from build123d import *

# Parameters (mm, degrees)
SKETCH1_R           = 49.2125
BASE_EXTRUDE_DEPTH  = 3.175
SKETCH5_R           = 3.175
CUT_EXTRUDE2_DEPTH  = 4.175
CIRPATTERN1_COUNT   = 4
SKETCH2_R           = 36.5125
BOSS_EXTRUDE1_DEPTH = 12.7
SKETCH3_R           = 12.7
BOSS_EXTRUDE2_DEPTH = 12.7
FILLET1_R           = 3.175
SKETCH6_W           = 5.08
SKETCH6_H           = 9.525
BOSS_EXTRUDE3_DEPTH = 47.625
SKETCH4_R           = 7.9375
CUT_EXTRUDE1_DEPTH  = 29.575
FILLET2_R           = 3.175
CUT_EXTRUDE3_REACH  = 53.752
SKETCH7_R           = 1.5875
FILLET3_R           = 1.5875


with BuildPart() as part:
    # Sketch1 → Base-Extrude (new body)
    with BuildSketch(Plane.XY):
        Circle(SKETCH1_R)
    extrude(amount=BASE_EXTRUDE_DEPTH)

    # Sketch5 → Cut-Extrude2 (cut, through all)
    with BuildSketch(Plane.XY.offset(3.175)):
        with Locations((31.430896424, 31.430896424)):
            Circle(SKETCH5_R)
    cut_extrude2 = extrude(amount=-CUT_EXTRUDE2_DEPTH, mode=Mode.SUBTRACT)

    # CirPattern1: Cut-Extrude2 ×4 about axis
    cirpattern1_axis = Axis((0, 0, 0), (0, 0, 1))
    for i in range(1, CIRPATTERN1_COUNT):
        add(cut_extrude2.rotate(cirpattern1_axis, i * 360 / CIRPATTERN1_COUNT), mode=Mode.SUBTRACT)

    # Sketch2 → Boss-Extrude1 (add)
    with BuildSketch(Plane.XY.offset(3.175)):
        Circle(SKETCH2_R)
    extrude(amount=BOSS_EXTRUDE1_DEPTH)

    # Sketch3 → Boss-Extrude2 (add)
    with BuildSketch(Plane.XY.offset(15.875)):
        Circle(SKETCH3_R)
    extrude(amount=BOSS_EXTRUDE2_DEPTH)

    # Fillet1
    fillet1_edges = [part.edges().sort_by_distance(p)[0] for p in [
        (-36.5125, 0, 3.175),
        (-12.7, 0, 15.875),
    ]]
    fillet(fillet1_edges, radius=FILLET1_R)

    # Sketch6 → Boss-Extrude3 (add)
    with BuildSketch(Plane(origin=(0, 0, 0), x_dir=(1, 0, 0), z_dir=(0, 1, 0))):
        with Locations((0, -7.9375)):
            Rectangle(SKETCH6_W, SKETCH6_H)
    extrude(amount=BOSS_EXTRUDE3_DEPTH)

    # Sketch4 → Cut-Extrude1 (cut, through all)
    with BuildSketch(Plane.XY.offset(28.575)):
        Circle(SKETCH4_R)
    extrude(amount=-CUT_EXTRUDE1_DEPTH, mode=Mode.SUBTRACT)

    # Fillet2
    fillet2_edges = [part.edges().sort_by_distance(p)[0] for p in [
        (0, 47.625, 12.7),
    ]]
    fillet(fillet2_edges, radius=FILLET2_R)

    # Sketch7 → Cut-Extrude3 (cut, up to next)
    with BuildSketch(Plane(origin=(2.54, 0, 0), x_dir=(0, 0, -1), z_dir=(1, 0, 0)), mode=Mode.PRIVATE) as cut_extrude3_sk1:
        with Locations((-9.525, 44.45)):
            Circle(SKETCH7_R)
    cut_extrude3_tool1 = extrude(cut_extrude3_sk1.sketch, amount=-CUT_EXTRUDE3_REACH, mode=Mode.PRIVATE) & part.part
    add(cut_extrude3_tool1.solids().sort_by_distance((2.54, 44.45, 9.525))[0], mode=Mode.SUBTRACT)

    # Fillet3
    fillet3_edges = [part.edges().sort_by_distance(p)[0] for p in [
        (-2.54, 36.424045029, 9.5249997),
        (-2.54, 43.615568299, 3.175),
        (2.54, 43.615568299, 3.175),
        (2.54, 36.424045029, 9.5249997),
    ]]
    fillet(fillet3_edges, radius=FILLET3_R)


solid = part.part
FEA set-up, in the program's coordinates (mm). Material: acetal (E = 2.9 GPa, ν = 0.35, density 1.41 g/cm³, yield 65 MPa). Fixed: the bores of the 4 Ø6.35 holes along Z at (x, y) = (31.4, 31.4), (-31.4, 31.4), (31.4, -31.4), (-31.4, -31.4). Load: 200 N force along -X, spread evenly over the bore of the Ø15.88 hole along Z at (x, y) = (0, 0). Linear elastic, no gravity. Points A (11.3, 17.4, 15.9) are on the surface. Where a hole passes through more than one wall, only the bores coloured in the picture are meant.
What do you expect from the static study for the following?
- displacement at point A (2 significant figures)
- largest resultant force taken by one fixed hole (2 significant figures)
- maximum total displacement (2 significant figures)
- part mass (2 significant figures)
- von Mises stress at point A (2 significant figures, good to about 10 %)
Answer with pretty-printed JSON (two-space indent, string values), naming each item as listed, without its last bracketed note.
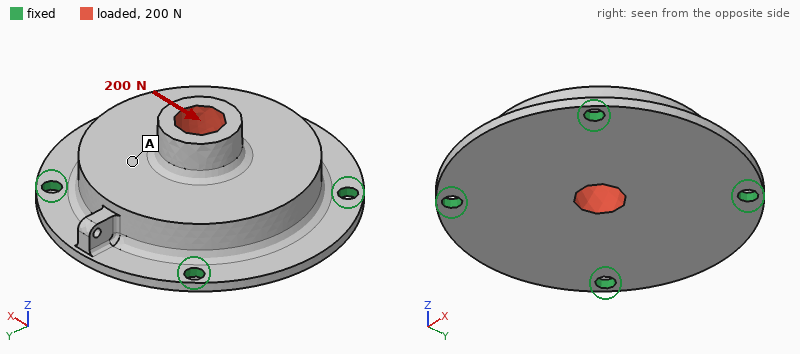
{
  "displacement at point A": "7.6 µm",
  "largest resultant force taken by one fixed hole": "58 N",
  "maximum total displacement": "17 µm",
  "part mass": "110 g",
  "von Mises stress at point A": "0.24 MPa"
}
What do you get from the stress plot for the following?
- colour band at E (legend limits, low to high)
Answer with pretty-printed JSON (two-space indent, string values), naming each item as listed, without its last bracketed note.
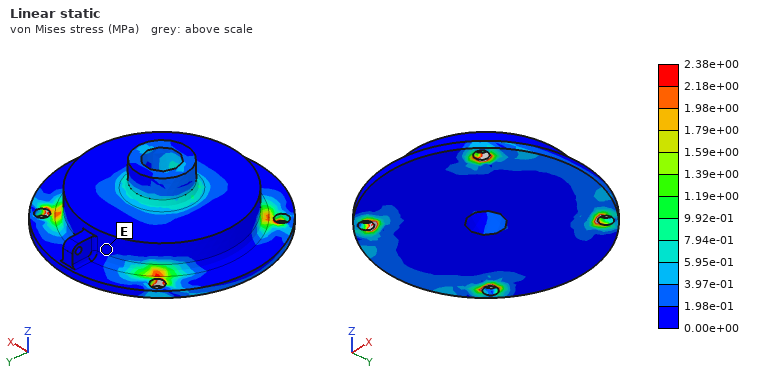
{
  "colour band at E": "0.00e+00 to 1.98e-01 MPa"
}
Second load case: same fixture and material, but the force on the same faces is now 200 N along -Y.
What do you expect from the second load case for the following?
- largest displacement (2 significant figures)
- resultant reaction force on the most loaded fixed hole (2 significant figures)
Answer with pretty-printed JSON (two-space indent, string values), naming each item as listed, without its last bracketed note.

{
  "largest displacement": "17 µm",
  "resultant reaction force on the most loaded fixed hole": "58 N"
}
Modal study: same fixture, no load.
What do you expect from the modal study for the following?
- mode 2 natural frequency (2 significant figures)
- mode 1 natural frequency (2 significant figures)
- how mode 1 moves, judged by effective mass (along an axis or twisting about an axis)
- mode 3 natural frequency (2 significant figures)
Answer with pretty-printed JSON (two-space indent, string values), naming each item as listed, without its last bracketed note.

{
  "mode 2 natural frequency": "2000 Hz",
  "mode 1 natural frequency": "1600 Hz",
  "how mode 1 moves, judged by effective mass": "along Z",
  "mode 3 natural frequency": "2100 Hz"
}
